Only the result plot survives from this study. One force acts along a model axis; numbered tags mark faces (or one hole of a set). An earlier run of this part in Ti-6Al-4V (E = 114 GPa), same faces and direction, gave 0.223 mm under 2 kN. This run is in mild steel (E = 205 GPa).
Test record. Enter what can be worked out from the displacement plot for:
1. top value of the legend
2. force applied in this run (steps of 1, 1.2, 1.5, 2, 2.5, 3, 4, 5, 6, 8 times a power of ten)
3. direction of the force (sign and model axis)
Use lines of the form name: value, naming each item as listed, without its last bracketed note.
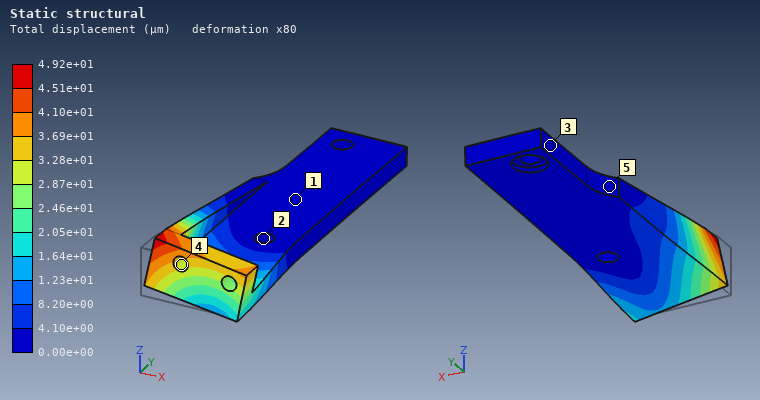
top value of the legend: 4.92e+01 µm
force applied in this run: 800 N
direction of the force: +X
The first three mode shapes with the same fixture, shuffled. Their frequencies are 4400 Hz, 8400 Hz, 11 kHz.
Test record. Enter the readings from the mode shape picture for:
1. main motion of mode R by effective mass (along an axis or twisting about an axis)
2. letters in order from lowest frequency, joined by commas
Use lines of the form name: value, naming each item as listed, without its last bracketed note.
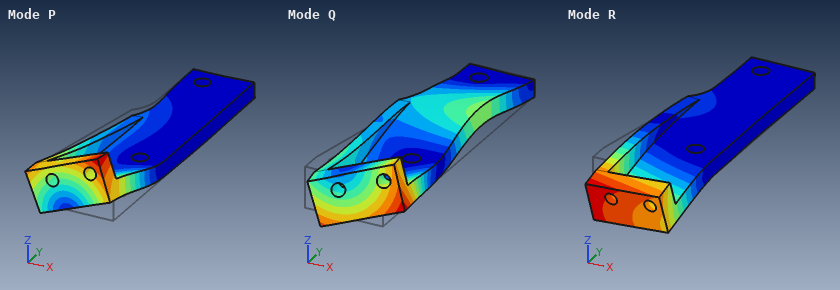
main motion of mode R by effective mass: along Z
letters in order from lowest frequency, joined by commas: R, P, Q
